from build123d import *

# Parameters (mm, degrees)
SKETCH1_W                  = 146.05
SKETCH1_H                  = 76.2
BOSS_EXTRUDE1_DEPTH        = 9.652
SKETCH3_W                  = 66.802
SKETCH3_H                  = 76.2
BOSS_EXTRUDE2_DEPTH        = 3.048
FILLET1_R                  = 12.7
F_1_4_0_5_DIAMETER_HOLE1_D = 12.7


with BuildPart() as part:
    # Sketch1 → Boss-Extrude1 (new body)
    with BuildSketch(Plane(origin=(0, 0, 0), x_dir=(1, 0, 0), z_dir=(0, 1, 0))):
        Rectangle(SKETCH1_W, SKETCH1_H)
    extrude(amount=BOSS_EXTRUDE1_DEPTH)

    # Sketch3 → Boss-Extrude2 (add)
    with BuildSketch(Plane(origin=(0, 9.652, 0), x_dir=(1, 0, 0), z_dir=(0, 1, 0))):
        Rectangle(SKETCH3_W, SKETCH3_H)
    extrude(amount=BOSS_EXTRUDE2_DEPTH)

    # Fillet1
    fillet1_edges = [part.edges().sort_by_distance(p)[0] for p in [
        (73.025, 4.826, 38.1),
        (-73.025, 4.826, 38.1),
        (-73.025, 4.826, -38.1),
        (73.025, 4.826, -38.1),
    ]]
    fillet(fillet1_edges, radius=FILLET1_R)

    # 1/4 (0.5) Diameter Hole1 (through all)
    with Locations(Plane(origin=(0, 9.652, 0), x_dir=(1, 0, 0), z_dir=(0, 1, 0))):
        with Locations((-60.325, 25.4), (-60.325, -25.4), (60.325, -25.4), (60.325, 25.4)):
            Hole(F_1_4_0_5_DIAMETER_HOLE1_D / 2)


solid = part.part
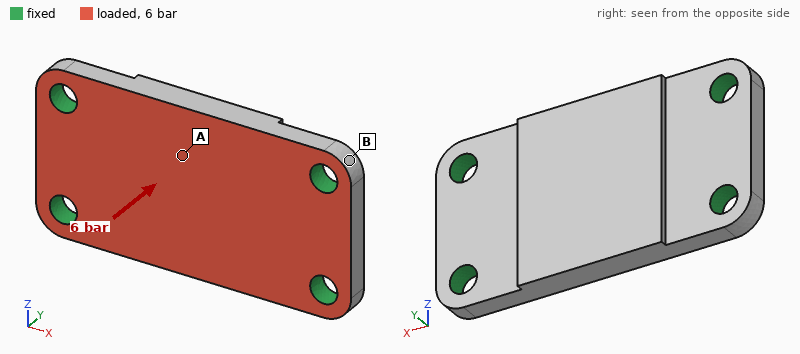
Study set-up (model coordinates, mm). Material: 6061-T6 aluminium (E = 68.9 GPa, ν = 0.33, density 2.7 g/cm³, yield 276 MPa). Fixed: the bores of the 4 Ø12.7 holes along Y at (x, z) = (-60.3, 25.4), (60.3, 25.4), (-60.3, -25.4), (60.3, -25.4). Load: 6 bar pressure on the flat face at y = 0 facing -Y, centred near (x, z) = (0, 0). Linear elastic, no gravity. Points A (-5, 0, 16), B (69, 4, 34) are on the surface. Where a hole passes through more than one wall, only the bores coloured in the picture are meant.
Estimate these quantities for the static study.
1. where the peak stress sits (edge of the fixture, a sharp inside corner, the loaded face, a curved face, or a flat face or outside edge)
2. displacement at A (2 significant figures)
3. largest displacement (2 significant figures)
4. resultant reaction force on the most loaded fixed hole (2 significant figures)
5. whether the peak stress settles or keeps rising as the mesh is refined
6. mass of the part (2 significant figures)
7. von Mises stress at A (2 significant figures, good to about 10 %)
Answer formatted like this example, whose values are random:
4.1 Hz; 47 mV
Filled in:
edge of the fixture; 37 µm; 41 µm; 1.7 kN; keeps rising; 320 g; 13 MPa
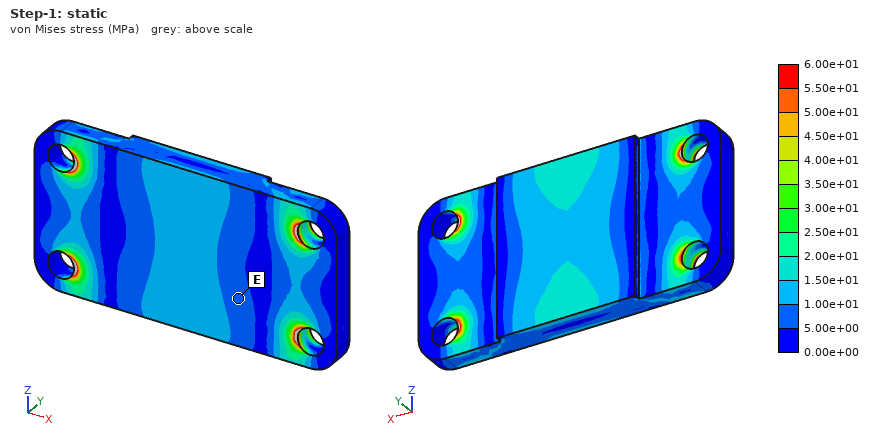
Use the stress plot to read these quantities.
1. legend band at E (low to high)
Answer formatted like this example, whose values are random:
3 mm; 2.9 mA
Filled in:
5.00e+00 to 1.00e+01 MPa
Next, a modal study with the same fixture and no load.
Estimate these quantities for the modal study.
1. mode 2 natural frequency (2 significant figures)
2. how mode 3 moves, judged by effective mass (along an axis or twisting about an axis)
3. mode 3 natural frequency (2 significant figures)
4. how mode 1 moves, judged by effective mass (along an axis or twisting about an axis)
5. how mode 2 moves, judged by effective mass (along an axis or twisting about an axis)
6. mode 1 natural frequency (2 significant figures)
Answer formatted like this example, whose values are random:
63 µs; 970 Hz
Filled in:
5300 Hz; twisting about Z; 10 kHz; along Y; twisting about X; 3900 Hz
